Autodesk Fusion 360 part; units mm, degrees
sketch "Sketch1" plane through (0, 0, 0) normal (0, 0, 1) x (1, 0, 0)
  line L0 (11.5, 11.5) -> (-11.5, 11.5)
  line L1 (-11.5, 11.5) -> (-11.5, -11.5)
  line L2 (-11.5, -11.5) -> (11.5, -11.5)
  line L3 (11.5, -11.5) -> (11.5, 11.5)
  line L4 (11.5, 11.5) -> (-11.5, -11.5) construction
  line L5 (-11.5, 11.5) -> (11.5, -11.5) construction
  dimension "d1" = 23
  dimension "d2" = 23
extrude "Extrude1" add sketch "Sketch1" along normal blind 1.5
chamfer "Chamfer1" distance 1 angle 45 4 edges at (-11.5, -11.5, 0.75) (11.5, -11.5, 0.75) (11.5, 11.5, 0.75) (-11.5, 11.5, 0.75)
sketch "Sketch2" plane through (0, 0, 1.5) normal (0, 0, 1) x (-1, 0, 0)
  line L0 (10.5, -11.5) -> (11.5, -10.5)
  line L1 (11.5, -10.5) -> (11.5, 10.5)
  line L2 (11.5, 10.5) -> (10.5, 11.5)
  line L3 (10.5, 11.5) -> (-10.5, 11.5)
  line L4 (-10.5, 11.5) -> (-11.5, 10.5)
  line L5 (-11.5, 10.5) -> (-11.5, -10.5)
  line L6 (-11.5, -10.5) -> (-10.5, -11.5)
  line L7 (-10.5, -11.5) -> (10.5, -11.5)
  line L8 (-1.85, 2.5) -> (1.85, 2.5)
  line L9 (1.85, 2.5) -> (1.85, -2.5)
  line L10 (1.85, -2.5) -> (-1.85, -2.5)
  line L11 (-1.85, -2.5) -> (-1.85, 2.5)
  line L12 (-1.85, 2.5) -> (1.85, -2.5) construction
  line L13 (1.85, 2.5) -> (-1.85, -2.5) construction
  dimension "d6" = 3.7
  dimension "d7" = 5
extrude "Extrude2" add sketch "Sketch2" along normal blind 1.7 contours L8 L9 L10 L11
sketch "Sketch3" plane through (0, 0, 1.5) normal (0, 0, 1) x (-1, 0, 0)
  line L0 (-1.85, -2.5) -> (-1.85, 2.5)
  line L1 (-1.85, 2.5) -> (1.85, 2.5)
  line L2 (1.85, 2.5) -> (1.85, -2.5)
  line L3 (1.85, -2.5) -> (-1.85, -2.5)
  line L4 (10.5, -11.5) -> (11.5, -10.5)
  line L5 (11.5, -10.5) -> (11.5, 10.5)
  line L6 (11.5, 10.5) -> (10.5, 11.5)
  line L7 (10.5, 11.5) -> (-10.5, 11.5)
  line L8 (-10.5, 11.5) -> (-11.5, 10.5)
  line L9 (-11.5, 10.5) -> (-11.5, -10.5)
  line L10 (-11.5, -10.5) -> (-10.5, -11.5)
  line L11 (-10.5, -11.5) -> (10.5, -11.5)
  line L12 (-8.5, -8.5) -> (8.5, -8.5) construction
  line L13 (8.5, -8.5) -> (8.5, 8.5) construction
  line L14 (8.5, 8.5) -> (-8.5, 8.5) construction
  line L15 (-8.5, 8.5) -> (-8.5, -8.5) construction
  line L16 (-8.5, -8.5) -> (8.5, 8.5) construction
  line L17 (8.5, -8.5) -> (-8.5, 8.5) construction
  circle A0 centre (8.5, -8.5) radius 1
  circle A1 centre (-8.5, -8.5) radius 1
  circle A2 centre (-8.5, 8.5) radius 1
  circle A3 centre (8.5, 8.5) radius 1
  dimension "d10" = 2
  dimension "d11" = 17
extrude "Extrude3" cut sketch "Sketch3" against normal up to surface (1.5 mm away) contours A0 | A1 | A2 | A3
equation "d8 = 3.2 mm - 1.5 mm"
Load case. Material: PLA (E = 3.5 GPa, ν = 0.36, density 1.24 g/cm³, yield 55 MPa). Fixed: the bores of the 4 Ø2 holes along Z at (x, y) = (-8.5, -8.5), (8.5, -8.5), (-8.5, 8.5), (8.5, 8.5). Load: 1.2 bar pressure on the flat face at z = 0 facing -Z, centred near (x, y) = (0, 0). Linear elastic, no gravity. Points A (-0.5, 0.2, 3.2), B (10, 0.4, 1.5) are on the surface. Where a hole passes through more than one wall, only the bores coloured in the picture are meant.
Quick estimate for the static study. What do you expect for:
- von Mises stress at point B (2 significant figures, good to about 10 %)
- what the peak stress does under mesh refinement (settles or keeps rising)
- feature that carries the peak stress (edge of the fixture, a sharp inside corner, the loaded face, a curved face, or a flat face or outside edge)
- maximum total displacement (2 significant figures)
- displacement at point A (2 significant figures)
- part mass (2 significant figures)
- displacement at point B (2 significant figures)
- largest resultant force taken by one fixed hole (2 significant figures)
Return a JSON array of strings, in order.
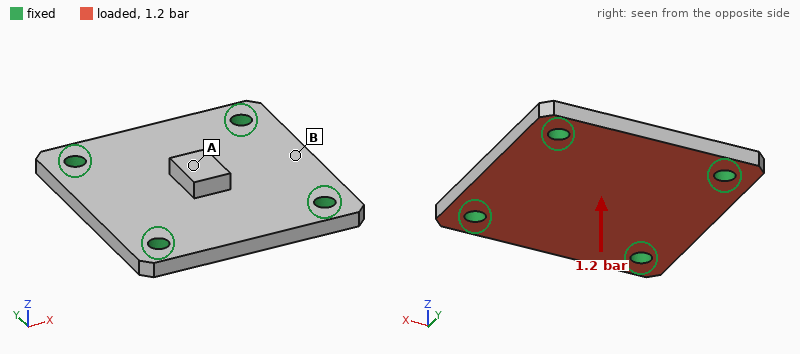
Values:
["3.8 MPa", "keeps rising", "edge of the fixture", "48 µm", "47 µm", "1.00 g", "25 µm", "15 N"]
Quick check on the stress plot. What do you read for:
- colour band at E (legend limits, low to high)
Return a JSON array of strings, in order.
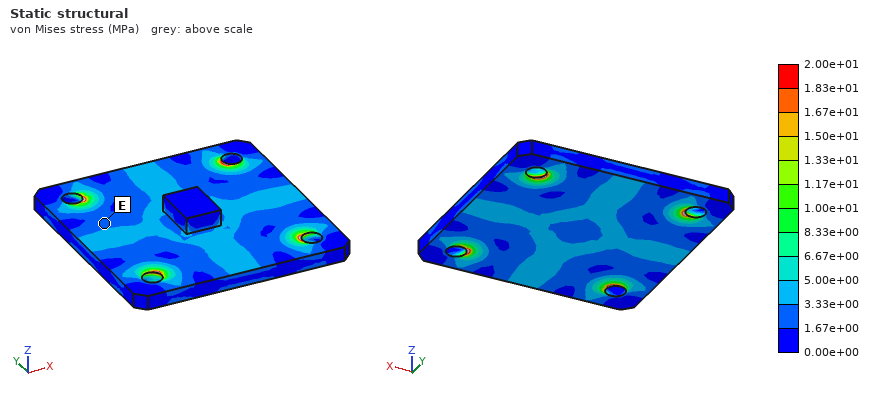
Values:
["1.67e+00 to 3.33e+00 MPa"]
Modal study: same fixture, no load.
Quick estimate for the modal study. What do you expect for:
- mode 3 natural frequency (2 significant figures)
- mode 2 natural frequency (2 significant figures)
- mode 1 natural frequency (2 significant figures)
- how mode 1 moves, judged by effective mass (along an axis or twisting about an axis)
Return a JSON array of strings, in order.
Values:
["10 kHz", "10 kHz", "6500 Hz", "along Z"]
